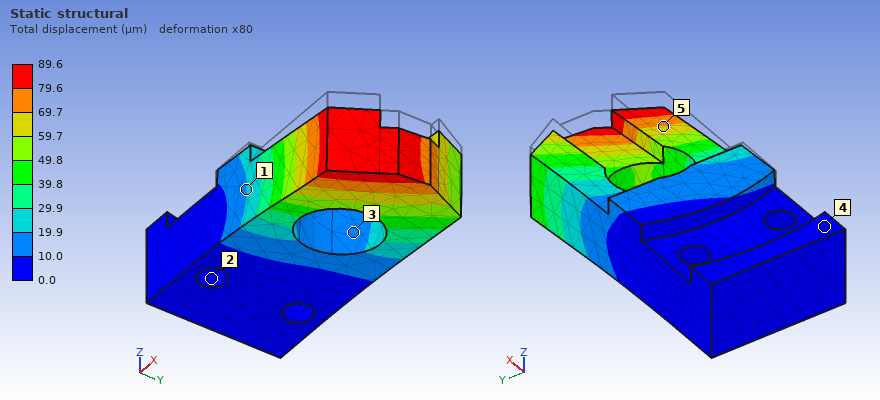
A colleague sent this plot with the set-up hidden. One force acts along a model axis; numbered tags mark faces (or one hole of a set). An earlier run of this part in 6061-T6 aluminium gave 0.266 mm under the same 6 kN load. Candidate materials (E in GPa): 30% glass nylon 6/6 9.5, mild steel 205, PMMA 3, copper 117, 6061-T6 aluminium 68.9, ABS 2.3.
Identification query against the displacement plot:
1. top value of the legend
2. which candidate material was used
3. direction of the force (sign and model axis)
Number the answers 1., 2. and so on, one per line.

1. 89.6 µm
2. mild steel
3. -Z
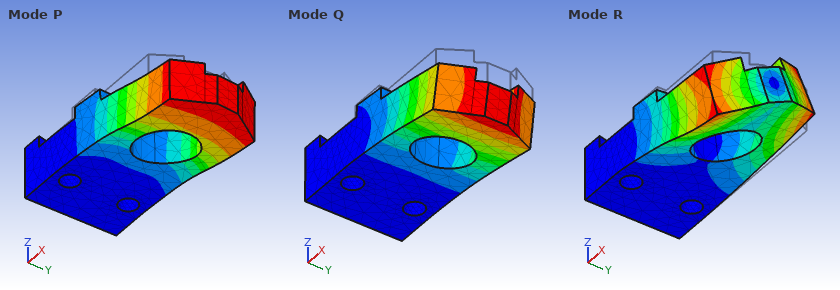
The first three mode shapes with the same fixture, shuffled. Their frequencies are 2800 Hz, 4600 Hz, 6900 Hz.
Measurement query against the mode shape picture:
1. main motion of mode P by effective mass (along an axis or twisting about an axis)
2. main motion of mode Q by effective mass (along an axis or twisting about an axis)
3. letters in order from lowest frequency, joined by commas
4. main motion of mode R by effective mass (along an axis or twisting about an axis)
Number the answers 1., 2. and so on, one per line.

1. along Y
2. along Z
3. Q, P, R
4. twisting about X
